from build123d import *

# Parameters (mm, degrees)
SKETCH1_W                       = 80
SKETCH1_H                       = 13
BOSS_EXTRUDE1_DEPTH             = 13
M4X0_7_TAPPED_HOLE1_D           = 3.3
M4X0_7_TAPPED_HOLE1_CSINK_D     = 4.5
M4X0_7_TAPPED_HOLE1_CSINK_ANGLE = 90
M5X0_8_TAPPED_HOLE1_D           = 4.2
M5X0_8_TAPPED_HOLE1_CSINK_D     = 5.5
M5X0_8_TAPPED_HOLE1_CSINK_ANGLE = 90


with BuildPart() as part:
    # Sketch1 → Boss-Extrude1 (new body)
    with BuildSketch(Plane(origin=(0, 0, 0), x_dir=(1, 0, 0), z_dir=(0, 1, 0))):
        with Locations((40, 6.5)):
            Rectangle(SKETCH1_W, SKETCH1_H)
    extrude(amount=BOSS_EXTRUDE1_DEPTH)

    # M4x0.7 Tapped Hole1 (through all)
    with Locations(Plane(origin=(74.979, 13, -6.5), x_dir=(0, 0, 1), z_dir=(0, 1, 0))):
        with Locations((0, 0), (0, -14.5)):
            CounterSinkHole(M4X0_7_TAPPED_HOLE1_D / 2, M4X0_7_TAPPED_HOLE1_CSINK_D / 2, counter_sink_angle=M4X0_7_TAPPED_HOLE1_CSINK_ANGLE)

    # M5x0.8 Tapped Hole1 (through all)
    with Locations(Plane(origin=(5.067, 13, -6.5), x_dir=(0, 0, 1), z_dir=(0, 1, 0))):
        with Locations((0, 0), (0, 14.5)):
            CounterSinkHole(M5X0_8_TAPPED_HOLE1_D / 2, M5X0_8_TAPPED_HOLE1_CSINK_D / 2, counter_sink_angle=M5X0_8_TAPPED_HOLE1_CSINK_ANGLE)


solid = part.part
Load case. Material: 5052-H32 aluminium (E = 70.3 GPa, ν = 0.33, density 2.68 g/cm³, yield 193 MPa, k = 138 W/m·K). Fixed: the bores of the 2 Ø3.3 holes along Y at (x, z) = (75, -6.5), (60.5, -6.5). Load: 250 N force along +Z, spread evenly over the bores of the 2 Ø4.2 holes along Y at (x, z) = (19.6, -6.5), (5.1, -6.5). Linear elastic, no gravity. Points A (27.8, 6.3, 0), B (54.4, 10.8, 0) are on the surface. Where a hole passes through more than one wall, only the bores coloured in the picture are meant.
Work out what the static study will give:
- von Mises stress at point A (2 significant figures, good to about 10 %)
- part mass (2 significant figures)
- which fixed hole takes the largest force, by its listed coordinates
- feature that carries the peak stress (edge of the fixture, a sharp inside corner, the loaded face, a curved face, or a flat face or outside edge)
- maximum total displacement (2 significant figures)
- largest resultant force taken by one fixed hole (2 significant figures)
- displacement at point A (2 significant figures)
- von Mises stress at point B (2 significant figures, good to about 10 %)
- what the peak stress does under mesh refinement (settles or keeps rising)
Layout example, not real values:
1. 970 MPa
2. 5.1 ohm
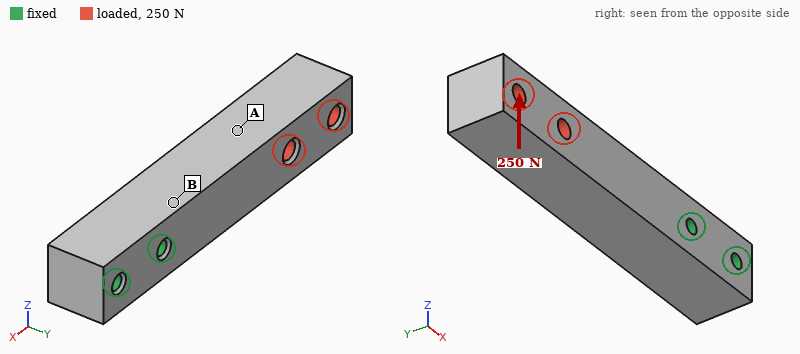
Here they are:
1. 11 MPa
2. 35 g
3. (60.5, -6.5)
4. edge of the fixture
5. 0.10 mm
6. 760 N
7. 0.045 mm
8. 29 MPa
9. keeps rising
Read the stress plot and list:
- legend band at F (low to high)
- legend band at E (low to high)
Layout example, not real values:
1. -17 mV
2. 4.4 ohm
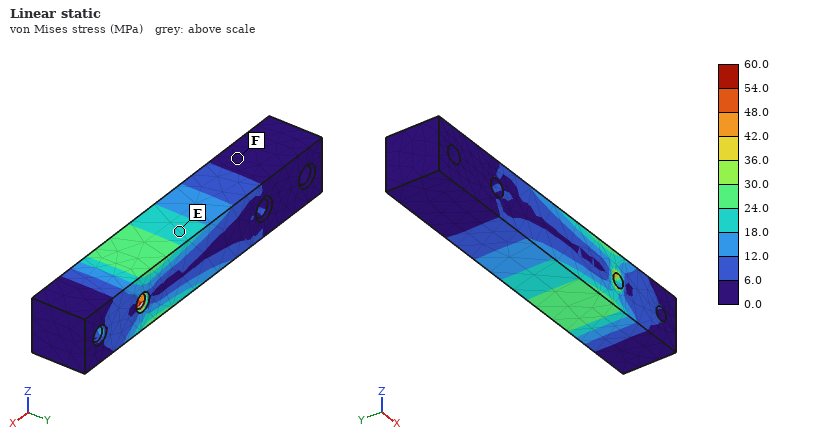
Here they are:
1. 0.0 to 6.0 MPa
2. 18.0 to 24.0 MPa
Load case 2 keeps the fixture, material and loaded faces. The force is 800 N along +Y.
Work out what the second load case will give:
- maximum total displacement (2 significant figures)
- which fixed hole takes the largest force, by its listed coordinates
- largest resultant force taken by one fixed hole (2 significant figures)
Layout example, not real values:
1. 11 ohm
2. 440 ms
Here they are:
1. 0.28 mm
2. (60.5, -6.5)
3. 1.3 kN
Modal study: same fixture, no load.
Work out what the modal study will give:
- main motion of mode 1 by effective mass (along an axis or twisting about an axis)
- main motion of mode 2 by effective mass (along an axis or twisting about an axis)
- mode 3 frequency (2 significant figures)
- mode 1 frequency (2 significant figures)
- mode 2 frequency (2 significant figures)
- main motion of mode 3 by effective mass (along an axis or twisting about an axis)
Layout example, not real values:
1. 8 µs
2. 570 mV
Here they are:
1. along Z
2. along Y
3. 12 kHz
4. 2600 Hz
5. 2900 Hz
6. twisting about X
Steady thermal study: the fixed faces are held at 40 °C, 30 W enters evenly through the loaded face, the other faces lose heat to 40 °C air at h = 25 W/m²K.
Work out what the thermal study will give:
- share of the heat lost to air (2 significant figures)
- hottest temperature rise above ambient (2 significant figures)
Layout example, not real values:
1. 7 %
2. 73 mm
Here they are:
1. 9.7 %
2. 61 K
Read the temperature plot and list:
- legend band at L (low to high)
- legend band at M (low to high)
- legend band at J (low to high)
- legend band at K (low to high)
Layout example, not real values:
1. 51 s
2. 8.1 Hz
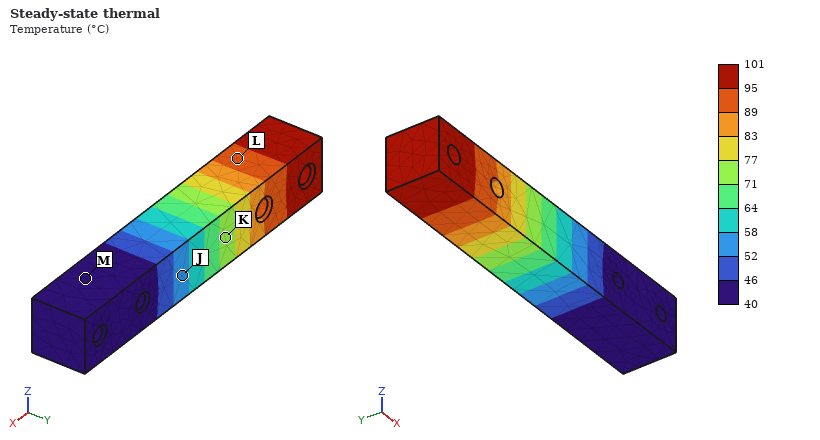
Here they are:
1. 89 to 95 °C
2. 40 to 46 °C
3. 52 to 58 °C
4. 71 to 77 °C
